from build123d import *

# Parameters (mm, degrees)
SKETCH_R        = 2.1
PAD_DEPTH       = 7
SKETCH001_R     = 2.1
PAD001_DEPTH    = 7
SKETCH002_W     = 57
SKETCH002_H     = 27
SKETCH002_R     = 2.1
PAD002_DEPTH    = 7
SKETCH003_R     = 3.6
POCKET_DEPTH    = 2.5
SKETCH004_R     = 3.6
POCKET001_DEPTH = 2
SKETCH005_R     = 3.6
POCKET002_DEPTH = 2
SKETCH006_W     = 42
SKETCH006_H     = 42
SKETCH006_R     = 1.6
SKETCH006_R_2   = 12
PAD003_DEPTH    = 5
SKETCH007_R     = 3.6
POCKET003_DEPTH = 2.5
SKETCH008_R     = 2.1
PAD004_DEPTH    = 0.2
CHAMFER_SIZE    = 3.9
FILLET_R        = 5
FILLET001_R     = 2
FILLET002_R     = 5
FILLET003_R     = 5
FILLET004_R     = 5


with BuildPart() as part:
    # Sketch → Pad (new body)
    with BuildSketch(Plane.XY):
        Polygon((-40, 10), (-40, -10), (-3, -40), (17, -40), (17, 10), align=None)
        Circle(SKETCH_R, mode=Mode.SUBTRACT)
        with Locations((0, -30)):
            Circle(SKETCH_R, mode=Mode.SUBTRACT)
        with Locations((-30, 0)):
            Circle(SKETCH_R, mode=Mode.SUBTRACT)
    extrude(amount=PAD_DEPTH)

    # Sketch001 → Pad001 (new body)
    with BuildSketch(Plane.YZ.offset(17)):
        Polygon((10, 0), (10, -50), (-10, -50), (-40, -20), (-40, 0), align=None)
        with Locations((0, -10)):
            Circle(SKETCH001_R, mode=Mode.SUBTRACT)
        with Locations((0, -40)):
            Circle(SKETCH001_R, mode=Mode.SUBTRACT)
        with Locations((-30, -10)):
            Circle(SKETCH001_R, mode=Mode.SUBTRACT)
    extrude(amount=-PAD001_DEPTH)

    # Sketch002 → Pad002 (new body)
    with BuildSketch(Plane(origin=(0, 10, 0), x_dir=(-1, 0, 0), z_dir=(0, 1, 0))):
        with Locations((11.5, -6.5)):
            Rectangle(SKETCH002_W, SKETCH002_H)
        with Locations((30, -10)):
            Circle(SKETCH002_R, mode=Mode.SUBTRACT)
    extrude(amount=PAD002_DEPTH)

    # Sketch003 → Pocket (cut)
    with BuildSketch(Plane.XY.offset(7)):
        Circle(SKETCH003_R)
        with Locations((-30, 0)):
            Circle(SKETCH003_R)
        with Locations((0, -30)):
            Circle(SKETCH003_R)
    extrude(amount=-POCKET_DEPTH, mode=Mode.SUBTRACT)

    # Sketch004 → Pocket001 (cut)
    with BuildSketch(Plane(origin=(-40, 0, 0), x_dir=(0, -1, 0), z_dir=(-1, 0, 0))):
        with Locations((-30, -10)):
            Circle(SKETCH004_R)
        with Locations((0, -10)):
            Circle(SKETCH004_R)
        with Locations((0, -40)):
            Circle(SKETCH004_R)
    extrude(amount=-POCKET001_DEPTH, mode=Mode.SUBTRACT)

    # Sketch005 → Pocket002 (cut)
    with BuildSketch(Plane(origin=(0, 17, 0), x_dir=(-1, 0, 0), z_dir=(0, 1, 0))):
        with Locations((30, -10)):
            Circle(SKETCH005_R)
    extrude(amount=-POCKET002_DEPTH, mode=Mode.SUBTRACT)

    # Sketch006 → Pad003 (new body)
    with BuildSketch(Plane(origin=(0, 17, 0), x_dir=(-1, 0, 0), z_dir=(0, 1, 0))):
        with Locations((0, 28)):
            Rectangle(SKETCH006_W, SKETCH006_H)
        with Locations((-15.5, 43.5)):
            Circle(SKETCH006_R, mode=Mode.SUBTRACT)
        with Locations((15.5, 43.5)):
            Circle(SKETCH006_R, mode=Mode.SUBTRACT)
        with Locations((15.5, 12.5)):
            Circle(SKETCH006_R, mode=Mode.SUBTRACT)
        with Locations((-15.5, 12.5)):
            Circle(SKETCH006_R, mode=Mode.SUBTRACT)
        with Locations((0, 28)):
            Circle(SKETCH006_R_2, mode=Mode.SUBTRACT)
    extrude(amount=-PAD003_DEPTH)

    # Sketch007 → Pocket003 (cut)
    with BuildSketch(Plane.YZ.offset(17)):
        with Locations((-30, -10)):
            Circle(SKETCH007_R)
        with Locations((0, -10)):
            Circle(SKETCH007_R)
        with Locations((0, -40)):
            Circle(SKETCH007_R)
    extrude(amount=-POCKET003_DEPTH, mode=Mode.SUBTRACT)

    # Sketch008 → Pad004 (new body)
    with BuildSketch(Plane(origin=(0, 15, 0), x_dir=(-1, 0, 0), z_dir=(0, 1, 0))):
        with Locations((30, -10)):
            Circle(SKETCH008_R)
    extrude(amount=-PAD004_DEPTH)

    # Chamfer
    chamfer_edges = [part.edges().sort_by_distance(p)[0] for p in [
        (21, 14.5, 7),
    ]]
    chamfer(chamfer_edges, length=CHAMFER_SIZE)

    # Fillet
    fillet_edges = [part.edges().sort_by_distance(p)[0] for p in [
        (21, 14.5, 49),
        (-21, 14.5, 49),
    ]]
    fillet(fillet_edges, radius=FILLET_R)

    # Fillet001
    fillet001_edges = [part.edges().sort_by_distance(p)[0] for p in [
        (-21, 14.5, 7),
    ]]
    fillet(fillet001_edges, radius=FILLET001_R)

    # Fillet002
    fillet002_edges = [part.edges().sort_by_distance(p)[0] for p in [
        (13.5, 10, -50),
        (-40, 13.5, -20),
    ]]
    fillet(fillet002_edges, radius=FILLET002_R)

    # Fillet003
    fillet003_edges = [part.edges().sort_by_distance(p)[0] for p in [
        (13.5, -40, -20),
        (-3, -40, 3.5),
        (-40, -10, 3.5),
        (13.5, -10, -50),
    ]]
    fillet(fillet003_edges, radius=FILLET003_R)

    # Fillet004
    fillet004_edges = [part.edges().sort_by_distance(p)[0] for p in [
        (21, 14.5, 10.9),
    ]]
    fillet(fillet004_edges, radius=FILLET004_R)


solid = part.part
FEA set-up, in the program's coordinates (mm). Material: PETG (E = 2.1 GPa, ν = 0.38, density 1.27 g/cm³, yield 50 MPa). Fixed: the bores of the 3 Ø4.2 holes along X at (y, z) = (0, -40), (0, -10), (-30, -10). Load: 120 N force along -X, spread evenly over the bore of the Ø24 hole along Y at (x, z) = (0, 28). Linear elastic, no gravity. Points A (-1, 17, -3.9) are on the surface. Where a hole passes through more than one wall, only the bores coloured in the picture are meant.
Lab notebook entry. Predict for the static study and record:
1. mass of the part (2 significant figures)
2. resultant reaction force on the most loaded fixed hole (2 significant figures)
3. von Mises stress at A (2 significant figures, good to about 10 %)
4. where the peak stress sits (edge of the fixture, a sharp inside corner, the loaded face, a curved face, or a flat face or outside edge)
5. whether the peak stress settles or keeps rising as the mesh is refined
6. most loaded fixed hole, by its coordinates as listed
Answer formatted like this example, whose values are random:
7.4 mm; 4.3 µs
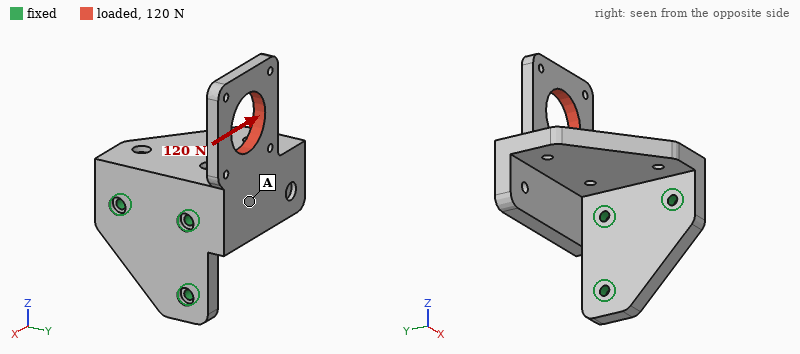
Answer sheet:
59 g; 270 N; 1.9 MPa; edge of the fixture; keeps rising; (0, -10)
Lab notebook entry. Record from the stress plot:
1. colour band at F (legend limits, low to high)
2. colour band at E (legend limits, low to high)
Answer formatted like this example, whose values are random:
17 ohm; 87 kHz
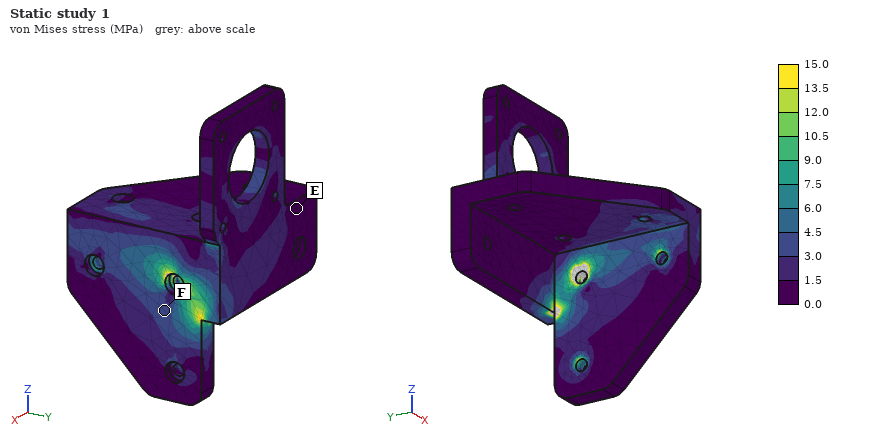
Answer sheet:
3.0 to 4.5 MPa; 0.0 to 1.5 MPa
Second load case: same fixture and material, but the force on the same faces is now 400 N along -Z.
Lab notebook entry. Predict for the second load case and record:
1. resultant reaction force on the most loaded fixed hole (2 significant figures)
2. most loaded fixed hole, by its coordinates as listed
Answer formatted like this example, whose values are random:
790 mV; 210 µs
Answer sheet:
470 N; (0, -10)
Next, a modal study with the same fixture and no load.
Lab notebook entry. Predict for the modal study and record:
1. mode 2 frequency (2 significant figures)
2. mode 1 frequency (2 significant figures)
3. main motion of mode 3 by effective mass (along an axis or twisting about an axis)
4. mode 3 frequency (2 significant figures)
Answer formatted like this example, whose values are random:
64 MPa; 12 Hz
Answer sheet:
450 Hz; 370 Hz; along Y; 780 Hz
